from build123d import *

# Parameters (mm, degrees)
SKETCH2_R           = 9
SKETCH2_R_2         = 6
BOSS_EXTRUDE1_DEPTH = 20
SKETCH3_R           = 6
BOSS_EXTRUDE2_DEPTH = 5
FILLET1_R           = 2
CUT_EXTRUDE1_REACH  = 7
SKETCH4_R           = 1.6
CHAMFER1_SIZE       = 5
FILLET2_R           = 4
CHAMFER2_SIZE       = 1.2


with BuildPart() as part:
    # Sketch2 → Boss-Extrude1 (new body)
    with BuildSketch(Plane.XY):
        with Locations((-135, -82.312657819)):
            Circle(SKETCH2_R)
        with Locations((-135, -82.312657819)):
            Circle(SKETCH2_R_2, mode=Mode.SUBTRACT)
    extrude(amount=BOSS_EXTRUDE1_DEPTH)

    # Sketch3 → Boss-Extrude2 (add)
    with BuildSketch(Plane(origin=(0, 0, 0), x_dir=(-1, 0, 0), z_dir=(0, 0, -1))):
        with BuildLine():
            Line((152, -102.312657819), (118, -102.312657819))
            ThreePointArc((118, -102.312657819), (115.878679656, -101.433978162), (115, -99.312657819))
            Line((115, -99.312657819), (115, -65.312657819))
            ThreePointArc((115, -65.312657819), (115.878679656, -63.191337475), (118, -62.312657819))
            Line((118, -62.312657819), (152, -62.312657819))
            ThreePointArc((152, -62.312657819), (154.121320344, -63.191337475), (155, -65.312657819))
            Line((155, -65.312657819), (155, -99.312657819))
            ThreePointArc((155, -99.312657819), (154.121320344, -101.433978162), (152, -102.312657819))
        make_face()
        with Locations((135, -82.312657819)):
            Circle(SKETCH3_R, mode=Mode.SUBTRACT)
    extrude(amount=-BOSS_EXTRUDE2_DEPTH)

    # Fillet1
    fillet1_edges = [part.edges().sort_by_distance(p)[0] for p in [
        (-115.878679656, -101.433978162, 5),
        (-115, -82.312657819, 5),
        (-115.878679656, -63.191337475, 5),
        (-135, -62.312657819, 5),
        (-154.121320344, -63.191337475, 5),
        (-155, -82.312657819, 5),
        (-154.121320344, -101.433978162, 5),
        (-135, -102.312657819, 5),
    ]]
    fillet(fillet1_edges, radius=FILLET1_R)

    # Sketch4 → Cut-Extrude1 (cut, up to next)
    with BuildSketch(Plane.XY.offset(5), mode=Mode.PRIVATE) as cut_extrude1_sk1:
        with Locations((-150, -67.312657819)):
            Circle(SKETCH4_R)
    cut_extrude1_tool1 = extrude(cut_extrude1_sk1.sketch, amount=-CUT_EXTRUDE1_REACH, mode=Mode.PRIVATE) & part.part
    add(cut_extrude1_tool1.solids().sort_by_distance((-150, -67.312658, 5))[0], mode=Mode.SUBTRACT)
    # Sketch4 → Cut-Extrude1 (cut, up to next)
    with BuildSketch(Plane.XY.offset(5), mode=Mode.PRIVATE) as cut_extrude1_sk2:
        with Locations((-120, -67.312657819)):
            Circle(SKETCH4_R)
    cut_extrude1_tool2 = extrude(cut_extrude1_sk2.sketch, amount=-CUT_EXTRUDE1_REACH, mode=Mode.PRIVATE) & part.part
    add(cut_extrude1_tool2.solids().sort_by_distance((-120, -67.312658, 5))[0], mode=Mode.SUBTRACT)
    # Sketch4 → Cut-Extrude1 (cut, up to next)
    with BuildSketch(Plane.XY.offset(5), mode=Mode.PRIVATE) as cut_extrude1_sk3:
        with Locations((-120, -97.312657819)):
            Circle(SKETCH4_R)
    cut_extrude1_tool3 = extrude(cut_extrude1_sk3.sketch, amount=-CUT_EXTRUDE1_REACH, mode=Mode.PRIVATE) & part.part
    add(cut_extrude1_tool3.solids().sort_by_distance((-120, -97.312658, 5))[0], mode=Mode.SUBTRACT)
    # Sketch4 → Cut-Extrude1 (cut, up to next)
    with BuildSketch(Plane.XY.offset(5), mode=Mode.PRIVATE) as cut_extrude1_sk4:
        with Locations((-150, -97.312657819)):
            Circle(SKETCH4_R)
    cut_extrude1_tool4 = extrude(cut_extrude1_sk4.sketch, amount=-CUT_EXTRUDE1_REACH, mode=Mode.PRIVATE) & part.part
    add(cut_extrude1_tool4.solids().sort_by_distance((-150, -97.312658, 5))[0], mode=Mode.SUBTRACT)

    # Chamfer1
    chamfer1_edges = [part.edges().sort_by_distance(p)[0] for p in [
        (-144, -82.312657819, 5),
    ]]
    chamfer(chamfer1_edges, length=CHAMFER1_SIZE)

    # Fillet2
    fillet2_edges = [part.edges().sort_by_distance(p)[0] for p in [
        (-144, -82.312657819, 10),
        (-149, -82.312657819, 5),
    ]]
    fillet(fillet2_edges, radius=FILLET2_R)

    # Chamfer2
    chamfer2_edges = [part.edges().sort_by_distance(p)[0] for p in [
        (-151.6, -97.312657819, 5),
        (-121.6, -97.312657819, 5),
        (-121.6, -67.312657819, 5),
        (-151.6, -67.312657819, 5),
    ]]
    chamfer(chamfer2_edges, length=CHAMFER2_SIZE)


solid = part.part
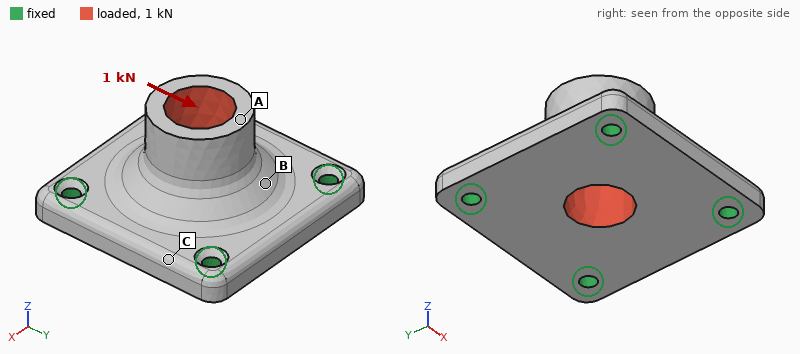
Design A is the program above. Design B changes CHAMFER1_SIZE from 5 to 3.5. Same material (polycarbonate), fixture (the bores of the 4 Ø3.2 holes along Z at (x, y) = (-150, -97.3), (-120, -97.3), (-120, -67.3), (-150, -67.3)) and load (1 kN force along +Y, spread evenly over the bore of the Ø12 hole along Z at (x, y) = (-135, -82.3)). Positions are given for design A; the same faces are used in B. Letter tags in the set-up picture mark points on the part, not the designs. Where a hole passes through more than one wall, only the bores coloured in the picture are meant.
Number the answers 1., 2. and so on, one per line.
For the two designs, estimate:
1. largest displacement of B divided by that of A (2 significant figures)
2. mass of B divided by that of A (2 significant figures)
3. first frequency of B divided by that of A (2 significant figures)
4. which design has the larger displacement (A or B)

1. 1.3
2. 0.96
3. 0.96
4. B
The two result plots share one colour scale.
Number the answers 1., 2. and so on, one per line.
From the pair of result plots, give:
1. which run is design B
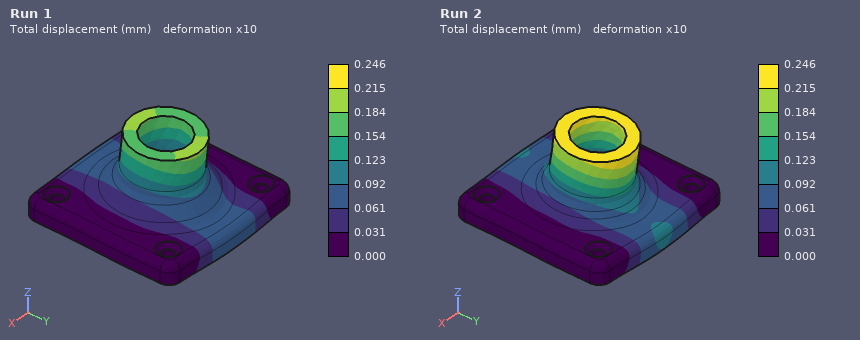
1. Run 2
